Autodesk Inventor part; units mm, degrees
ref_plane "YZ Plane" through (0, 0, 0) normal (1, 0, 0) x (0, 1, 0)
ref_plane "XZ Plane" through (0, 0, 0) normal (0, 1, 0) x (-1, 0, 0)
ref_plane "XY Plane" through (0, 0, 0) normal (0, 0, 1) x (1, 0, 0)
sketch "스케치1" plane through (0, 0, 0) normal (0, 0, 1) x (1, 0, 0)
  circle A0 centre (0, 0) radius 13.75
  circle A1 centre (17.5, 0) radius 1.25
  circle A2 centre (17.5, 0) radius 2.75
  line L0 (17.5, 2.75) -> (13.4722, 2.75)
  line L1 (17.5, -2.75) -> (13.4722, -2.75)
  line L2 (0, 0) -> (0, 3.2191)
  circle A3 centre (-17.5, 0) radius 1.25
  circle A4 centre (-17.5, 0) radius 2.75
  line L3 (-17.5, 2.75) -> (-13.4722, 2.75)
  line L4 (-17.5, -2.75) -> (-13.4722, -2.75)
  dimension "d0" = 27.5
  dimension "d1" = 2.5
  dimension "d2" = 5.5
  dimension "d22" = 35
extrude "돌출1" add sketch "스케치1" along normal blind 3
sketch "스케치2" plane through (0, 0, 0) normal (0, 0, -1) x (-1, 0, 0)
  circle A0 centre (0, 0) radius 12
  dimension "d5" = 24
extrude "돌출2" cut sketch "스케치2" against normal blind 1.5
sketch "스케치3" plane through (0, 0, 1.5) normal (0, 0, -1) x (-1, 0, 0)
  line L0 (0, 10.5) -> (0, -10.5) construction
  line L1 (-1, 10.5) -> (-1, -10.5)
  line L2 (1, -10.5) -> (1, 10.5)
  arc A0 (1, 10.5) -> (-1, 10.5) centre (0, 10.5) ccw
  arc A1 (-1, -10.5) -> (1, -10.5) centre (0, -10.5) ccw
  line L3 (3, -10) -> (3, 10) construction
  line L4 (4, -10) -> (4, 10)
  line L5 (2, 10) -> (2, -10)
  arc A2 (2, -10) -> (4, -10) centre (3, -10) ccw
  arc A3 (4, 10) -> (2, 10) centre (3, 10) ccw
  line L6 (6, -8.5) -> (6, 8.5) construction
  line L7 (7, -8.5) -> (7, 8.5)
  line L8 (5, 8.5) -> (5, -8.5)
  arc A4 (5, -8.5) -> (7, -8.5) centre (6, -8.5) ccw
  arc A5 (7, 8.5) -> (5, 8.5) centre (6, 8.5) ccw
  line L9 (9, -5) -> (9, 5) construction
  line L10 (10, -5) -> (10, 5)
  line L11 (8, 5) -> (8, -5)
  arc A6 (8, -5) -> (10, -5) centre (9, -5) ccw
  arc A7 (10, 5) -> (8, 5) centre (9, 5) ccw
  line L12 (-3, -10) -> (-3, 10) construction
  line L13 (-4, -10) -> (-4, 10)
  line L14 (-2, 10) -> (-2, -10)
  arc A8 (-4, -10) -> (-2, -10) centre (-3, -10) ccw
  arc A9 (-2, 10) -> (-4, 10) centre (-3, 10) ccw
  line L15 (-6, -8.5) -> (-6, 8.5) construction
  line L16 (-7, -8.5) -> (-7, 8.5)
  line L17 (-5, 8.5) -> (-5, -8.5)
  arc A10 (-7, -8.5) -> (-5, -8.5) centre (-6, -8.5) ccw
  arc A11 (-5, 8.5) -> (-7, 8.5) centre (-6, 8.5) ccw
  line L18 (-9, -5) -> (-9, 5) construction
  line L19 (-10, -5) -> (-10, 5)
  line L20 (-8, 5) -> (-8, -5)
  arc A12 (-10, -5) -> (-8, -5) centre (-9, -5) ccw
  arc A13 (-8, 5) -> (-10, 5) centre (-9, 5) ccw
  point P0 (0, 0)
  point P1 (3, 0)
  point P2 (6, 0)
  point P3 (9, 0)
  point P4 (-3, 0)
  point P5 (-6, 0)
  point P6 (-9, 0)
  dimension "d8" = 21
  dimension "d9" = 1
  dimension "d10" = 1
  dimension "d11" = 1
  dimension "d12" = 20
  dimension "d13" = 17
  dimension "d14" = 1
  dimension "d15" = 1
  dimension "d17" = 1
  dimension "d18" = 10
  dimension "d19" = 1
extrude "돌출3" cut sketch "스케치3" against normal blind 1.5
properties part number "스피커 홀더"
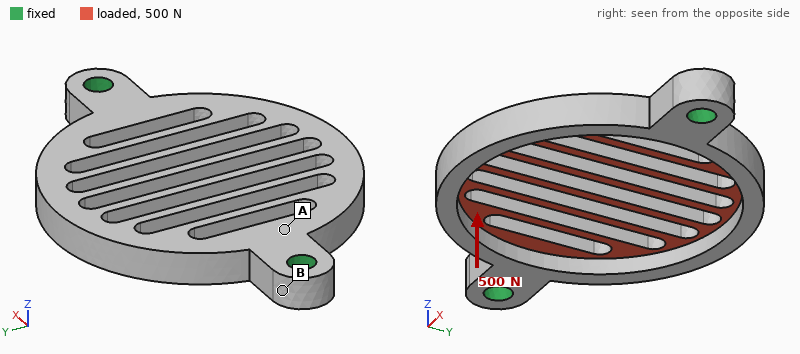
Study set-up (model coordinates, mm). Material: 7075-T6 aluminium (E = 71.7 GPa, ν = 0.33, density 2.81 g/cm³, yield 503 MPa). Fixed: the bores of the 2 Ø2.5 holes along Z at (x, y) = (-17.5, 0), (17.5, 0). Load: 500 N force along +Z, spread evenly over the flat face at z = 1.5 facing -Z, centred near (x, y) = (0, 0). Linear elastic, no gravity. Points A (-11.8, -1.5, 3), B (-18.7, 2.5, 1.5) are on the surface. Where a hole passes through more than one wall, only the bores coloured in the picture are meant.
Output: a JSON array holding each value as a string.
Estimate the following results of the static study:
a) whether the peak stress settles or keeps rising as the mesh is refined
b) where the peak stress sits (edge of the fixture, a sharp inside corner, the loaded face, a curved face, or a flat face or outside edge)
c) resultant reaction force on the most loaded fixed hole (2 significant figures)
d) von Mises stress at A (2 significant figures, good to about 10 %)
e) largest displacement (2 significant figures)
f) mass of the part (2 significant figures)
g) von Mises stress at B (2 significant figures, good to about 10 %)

["keeps rising", "edge of the fixture", "260 N", "110 MPa", "0.25 mm", "2.5 g", "31 MPa"]
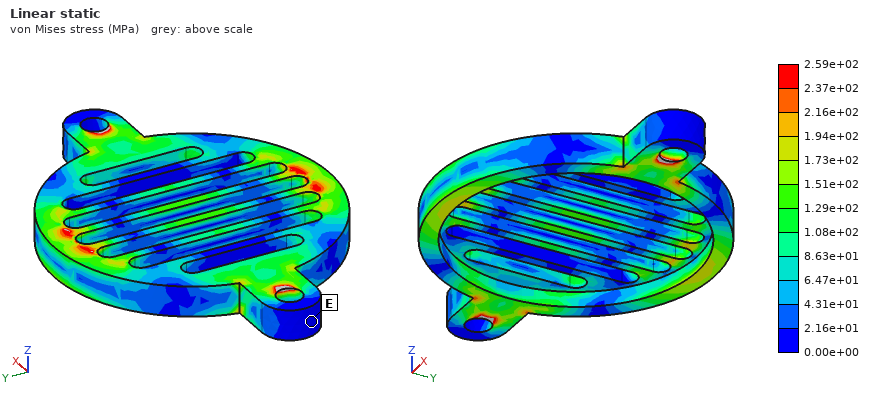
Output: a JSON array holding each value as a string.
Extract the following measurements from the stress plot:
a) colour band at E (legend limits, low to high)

["0.00e+00 to 2.16e+01 MPa"]
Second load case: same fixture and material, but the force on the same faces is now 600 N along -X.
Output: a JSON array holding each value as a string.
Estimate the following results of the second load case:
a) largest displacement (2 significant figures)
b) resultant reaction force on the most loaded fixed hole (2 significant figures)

["0.24 mm", "300 N"]
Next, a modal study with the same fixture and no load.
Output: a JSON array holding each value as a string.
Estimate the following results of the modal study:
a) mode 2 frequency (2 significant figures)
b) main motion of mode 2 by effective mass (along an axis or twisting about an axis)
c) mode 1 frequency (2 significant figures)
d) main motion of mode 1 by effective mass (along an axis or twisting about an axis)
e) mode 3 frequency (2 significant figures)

["7100 Hz", "along Z", "6200 Hz", "twisting about X", "10 kHz"]
